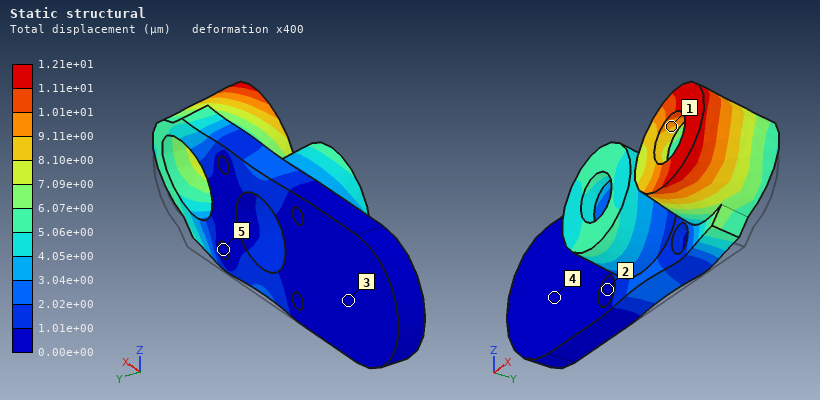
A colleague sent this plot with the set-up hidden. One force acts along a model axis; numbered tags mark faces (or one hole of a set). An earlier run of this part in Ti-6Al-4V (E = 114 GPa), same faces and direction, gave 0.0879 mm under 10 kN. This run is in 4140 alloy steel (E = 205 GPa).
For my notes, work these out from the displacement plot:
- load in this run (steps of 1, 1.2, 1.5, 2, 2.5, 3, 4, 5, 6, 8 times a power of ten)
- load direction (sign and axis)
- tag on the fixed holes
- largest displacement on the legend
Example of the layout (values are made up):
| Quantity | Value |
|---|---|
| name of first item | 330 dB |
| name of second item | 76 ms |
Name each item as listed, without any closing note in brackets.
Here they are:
| Quantity | Value |
|---|---|
| load in this run | 2.5 kN |
| load direction | +Z |
| tag on the fixed holes | 5 |
| largest displacement on the legend | 1.21e+01 µm |
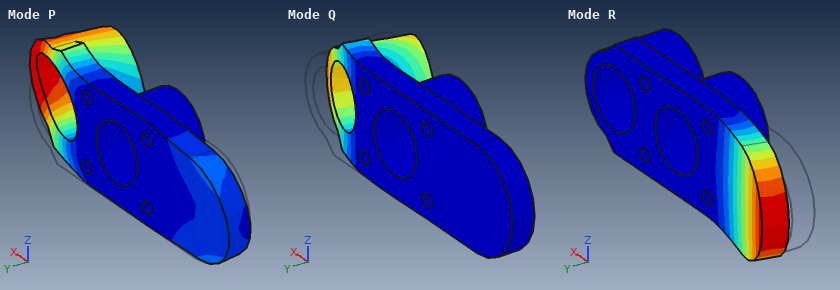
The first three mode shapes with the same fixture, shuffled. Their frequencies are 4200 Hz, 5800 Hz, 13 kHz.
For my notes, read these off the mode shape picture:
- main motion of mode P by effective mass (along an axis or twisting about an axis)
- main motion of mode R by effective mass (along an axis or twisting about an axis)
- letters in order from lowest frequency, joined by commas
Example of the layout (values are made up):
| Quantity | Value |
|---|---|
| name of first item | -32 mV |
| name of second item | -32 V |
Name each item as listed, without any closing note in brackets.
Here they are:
| Quantity | Value |
|---|---|
| main motion of mode P by effective mass | along Z |
| main motion of mode R by effective mass | along Y |
| letters in order from lowest frequency, joined by commas | R, Q, P |
